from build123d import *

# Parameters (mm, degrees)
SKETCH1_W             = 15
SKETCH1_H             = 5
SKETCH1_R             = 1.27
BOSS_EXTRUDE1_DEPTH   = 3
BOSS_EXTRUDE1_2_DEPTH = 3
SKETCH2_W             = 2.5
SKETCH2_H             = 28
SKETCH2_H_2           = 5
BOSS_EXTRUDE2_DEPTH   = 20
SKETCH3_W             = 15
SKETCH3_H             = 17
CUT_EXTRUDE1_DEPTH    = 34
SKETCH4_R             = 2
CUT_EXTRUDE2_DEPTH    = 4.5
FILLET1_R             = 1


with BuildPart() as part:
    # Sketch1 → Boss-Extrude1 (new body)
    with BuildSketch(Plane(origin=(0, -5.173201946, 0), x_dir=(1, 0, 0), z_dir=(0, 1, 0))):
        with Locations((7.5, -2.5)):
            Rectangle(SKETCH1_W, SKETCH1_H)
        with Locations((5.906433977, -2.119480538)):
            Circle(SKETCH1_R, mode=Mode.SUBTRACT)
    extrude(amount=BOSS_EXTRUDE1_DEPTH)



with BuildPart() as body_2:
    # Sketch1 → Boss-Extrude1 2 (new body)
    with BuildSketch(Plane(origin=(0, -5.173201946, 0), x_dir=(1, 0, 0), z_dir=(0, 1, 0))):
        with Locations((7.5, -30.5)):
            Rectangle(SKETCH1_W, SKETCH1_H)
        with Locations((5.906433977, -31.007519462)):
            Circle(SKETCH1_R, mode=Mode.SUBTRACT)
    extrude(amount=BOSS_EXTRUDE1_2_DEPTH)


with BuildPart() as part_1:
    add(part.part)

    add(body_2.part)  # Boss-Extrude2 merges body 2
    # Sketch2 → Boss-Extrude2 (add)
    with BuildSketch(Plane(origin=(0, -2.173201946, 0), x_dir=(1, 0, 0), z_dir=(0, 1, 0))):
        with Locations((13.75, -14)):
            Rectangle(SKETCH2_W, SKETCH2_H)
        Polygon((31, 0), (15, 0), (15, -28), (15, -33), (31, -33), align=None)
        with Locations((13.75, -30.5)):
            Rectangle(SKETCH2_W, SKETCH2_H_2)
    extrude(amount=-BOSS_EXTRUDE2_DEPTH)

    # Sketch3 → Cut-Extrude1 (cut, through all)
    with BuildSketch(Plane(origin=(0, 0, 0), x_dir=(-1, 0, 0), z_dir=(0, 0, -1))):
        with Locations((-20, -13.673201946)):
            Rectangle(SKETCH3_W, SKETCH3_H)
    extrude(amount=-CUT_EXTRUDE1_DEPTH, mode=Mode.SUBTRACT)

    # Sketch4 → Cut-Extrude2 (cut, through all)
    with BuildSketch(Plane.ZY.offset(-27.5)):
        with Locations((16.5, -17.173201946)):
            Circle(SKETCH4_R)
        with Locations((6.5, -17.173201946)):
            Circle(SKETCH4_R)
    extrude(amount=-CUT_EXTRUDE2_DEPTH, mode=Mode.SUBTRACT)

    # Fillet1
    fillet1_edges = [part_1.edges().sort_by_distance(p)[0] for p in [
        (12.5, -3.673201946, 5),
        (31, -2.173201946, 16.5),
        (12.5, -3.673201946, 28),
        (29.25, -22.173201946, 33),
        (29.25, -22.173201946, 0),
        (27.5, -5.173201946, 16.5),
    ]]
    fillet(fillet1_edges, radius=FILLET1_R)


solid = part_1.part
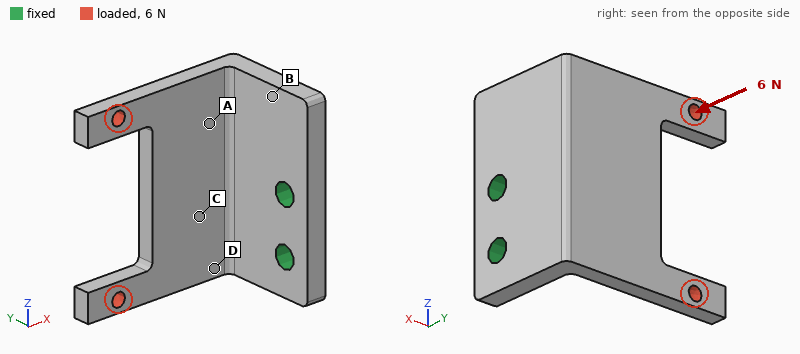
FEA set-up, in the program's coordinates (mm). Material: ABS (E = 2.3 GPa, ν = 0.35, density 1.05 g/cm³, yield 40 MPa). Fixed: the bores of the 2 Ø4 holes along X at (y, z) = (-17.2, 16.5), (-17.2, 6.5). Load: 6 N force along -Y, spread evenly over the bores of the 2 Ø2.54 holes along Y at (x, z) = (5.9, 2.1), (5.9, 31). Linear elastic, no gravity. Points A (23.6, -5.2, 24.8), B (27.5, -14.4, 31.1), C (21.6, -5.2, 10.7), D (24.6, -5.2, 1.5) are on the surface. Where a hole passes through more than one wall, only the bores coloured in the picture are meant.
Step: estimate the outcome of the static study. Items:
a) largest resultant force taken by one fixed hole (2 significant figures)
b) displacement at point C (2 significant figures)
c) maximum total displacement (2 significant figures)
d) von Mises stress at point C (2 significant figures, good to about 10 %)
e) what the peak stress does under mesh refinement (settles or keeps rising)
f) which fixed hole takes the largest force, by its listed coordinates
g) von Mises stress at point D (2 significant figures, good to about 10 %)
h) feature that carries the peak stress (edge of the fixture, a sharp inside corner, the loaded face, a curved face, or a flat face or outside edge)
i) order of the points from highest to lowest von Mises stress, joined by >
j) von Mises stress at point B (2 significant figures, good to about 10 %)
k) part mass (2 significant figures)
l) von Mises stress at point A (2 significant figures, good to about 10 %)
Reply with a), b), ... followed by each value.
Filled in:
a) 5.2 N
b) 0.069 mm
c) 0.45 mm
d) 1.6 MPa
e) keeps rising
f) (-17.2, 16.5)
g) 2.4 MPa
h) edge of the fixture
i) D > A > C > B
j) 1.1 MPa
k) 4.3 g
l) 1.9 MPa
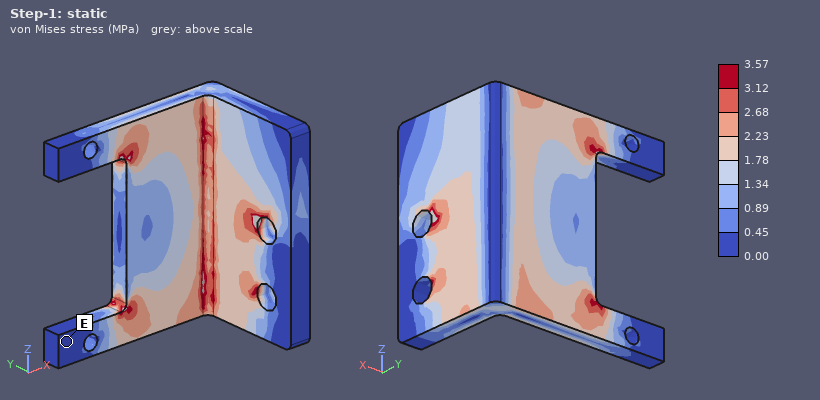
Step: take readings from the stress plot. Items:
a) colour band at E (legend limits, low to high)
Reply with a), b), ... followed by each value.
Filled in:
a) 0.00 to 0.45 MPa
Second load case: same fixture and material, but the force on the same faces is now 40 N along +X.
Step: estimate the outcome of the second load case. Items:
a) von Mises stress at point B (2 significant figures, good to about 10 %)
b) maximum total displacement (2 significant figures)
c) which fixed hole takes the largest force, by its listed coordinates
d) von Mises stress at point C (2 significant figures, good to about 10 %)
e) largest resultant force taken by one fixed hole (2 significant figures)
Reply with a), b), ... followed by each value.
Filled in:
a) 2.1 MPa
b) 0.50 mm
c) (-17.2, 16.5)
d) 0.74 MPa
e) 32 N
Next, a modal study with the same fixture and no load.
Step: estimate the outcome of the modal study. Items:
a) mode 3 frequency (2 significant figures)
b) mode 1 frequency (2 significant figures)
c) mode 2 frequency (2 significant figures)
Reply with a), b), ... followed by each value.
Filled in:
a) 1600 Hz
b) 880 Hz
c) 1300 Hz
